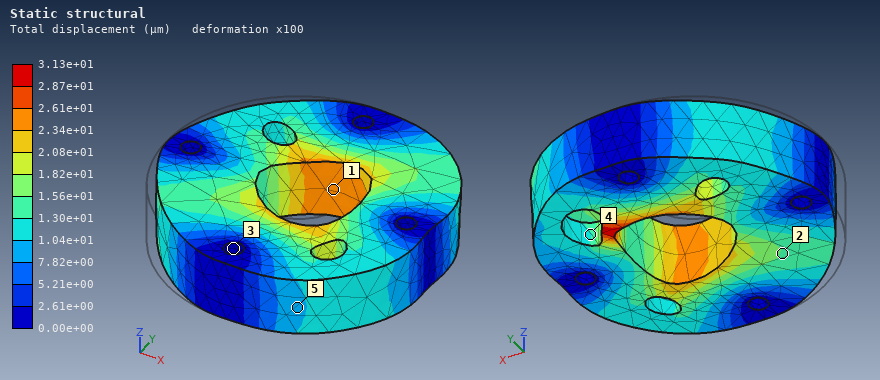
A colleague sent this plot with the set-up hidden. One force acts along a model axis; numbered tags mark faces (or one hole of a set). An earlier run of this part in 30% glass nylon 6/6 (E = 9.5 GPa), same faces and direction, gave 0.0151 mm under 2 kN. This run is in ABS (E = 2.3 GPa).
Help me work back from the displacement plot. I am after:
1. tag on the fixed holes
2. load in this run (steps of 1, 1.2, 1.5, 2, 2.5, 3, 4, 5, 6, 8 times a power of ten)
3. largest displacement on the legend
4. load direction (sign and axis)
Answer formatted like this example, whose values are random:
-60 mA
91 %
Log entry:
3
1 kN
3.13e+01 µm
+X
